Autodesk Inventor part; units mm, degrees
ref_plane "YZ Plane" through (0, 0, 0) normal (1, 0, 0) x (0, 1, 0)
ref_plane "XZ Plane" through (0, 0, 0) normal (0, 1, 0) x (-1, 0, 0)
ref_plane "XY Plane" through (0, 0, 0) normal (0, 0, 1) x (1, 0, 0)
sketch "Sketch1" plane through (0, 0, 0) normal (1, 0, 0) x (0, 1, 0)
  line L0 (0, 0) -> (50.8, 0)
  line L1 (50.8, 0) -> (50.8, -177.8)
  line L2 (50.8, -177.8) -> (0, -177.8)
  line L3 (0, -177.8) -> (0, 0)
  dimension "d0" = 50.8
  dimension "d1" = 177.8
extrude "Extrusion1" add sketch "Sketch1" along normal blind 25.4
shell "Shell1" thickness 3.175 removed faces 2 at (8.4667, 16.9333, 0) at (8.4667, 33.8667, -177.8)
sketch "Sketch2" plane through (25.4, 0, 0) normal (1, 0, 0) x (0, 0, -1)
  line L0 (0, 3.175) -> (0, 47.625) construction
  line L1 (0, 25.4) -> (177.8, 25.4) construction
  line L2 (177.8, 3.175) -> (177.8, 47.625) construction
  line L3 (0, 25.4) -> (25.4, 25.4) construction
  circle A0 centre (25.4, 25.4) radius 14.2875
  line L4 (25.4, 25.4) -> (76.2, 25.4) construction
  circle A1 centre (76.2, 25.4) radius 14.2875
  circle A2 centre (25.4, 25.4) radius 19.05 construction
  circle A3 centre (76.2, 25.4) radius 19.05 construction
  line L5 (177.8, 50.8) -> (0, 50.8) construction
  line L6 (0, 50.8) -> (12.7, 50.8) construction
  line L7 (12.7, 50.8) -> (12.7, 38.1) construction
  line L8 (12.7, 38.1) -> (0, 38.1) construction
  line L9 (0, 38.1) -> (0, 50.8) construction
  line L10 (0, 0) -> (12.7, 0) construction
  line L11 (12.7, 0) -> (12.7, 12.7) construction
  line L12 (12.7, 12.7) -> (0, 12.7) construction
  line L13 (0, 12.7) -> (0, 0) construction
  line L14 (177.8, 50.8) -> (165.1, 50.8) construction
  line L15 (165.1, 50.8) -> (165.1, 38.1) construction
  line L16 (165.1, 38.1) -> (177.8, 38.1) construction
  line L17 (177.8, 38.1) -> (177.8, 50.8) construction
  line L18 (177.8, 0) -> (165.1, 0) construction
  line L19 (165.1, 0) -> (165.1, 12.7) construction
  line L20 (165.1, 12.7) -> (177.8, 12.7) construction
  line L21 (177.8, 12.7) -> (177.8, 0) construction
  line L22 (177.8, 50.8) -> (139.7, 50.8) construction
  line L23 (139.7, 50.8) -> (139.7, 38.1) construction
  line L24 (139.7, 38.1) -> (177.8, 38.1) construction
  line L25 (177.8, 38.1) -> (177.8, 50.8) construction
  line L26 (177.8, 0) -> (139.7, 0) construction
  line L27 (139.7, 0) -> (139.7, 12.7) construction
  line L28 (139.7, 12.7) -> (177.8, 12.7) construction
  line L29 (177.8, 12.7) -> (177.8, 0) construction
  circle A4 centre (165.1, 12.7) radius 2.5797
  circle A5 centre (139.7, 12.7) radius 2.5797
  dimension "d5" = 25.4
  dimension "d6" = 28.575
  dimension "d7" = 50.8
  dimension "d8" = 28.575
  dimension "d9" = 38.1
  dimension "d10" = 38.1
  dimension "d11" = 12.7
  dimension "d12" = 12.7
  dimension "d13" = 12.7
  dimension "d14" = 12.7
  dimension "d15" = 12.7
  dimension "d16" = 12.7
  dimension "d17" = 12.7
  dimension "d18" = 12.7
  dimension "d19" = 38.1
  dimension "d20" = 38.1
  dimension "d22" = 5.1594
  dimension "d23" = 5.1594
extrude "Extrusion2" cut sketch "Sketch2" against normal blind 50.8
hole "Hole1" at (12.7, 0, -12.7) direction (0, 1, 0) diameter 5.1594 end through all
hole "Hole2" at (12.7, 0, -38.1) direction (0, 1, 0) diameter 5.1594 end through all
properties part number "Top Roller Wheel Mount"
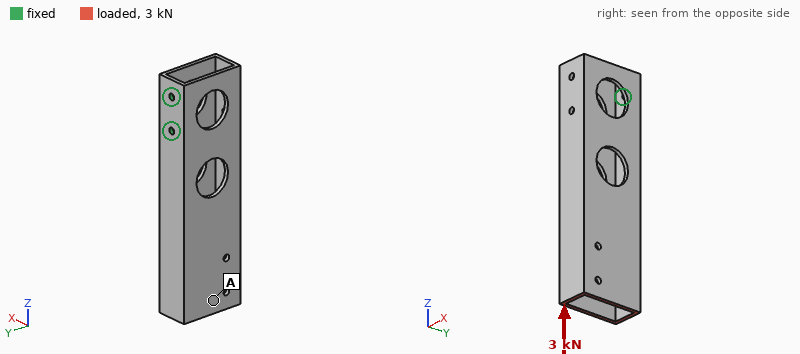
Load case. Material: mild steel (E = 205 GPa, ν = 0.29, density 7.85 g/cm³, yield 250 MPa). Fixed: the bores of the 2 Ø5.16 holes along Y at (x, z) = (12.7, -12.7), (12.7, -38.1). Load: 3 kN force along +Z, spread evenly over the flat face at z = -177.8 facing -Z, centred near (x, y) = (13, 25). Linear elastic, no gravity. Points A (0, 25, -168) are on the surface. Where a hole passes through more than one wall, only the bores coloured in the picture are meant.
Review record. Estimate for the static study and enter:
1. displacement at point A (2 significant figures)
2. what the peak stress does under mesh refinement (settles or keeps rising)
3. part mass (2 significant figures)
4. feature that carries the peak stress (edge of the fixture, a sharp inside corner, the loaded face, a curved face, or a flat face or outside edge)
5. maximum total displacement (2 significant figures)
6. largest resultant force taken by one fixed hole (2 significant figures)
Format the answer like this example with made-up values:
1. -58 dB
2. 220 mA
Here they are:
1. 0.25 mm
2. keeps rising
3. 550 g
4. edge of the fixture
5. 0.28 mm
6. 2.9 kN
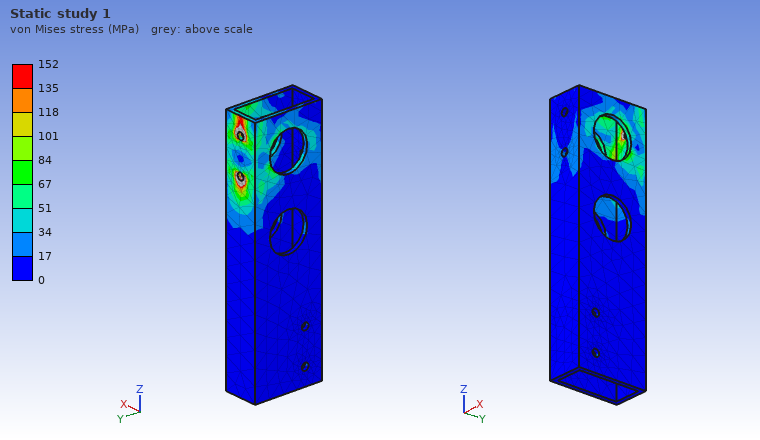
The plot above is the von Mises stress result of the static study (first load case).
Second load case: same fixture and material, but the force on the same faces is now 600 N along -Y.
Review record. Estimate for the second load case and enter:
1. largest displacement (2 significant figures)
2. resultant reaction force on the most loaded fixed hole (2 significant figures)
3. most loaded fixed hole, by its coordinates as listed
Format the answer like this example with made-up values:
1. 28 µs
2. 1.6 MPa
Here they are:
1. 0.38 mm
2. 3.3 kN
3. (12.7, -38.1)
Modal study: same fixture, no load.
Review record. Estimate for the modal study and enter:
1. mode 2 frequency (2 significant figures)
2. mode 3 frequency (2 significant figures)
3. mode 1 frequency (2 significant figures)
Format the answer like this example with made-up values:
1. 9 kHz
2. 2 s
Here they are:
1. 490 Hz
2. 840 Hz
3. 480 Hz
